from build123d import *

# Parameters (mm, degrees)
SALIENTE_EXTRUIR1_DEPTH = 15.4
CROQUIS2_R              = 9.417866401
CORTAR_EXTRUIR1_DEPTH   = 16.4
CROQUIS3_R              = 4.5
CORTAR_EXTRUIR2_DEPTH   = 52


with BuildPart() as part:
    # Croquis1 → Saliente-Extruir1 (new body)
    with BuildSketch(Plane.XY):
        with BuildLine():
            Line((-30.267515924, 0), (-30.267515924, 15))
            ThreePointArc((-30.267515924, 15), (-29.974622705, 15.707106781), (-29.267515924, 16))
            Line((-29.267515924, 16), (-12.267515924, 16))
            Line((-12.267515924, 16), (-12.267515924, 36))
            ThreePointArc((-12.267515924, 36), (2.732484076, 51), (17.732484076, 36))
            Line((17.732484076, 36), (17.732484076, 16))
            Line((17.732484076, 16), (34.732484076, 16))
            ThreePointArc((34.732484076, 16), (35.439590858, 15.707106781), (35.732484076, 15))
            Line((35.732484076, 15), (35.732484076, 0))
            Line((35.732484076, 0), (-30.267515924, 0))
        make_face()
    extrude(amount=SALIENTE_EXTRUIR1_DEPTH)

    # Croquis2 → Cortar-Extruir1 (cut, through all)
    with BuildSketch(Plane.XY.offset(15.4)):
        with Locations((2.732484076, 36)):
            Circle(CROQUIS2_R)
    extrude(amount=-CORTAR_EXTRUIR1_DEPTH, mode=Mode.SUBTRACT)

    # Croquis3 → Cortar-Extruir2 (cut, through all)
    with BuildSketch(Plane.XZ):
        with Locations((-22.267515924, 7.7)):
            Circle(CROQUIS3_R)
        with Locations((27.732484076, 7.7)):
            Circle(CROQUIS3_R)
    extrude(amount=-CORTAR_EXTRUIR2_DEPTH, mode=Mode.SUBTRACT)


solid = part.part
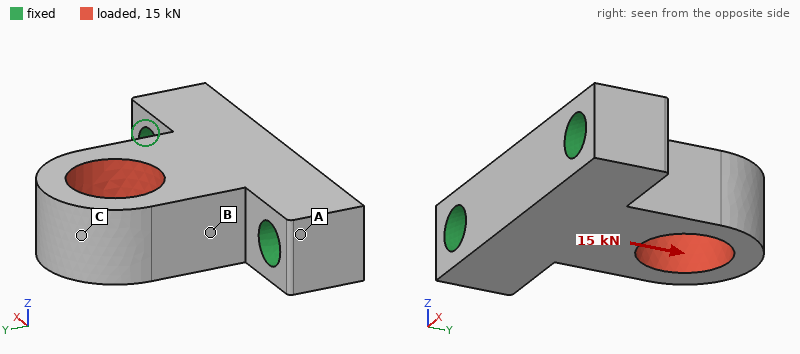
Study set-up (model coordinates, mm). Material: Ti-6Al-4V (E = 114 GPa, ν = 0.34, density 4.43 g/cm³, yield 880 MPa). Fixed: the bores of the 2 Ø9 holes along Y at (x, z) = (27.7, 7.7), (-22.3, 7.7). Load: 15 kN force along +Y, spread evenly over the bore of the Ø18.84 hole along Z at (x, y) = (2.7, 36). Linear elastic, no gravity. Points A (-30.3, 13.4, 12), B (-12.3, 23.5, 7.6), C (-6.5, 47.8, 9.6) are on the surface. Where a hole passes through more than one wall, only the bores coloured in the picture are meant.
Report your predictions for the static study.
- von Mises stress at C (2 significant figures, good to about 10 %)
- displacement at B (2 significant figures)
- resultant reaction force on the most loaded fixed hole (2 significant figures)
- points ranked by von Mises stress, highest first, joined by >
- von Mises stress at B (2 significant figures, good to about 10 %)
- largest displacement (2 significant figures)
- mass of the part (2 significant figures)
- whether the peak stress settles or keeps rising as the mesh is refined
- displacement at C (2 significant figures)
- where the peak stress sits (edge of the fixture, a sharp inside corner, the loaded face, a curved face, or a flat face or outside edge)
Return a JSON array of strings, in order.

["29 MPa", "15 µm", "7.8 kN", "B > C > A", "71 MPa", "36 µm", "110 g", "keeps rising", "25 µm", "edge of the fixture"]
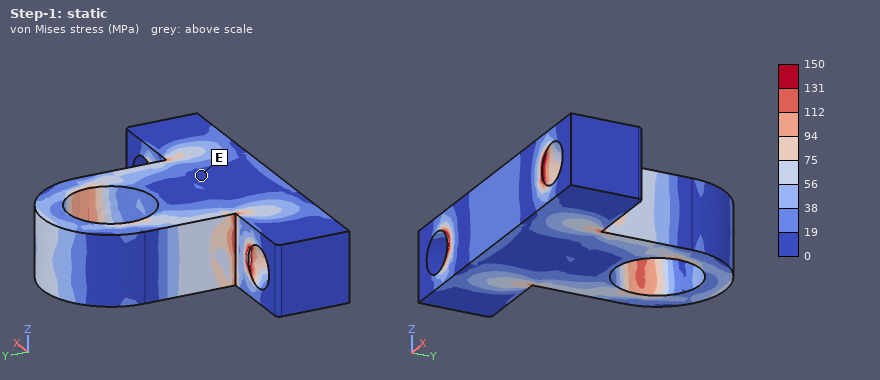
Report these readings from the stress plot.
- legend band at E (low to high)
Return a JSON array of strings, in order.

["0 to 19 MPa"]
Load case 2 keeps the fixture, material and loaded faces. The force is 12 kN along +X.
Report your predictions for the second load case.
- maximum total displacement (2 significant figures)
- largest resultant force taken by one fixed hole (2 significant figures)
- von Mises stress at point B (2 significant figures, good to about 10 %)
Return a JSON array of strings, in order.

["0.12 mm", "10 kN", "150 MPa"]
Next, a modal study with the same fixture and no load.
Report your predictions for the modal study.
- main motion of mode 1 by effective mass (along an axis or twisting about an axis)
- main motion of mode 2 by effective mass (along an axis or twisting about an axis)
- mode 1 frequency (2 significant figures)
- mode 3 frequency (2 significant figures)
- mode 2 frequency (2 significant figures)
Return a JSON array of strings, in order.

["along Z", "along X", "5800 Hz", "15 kHz", "10 kHz"]
